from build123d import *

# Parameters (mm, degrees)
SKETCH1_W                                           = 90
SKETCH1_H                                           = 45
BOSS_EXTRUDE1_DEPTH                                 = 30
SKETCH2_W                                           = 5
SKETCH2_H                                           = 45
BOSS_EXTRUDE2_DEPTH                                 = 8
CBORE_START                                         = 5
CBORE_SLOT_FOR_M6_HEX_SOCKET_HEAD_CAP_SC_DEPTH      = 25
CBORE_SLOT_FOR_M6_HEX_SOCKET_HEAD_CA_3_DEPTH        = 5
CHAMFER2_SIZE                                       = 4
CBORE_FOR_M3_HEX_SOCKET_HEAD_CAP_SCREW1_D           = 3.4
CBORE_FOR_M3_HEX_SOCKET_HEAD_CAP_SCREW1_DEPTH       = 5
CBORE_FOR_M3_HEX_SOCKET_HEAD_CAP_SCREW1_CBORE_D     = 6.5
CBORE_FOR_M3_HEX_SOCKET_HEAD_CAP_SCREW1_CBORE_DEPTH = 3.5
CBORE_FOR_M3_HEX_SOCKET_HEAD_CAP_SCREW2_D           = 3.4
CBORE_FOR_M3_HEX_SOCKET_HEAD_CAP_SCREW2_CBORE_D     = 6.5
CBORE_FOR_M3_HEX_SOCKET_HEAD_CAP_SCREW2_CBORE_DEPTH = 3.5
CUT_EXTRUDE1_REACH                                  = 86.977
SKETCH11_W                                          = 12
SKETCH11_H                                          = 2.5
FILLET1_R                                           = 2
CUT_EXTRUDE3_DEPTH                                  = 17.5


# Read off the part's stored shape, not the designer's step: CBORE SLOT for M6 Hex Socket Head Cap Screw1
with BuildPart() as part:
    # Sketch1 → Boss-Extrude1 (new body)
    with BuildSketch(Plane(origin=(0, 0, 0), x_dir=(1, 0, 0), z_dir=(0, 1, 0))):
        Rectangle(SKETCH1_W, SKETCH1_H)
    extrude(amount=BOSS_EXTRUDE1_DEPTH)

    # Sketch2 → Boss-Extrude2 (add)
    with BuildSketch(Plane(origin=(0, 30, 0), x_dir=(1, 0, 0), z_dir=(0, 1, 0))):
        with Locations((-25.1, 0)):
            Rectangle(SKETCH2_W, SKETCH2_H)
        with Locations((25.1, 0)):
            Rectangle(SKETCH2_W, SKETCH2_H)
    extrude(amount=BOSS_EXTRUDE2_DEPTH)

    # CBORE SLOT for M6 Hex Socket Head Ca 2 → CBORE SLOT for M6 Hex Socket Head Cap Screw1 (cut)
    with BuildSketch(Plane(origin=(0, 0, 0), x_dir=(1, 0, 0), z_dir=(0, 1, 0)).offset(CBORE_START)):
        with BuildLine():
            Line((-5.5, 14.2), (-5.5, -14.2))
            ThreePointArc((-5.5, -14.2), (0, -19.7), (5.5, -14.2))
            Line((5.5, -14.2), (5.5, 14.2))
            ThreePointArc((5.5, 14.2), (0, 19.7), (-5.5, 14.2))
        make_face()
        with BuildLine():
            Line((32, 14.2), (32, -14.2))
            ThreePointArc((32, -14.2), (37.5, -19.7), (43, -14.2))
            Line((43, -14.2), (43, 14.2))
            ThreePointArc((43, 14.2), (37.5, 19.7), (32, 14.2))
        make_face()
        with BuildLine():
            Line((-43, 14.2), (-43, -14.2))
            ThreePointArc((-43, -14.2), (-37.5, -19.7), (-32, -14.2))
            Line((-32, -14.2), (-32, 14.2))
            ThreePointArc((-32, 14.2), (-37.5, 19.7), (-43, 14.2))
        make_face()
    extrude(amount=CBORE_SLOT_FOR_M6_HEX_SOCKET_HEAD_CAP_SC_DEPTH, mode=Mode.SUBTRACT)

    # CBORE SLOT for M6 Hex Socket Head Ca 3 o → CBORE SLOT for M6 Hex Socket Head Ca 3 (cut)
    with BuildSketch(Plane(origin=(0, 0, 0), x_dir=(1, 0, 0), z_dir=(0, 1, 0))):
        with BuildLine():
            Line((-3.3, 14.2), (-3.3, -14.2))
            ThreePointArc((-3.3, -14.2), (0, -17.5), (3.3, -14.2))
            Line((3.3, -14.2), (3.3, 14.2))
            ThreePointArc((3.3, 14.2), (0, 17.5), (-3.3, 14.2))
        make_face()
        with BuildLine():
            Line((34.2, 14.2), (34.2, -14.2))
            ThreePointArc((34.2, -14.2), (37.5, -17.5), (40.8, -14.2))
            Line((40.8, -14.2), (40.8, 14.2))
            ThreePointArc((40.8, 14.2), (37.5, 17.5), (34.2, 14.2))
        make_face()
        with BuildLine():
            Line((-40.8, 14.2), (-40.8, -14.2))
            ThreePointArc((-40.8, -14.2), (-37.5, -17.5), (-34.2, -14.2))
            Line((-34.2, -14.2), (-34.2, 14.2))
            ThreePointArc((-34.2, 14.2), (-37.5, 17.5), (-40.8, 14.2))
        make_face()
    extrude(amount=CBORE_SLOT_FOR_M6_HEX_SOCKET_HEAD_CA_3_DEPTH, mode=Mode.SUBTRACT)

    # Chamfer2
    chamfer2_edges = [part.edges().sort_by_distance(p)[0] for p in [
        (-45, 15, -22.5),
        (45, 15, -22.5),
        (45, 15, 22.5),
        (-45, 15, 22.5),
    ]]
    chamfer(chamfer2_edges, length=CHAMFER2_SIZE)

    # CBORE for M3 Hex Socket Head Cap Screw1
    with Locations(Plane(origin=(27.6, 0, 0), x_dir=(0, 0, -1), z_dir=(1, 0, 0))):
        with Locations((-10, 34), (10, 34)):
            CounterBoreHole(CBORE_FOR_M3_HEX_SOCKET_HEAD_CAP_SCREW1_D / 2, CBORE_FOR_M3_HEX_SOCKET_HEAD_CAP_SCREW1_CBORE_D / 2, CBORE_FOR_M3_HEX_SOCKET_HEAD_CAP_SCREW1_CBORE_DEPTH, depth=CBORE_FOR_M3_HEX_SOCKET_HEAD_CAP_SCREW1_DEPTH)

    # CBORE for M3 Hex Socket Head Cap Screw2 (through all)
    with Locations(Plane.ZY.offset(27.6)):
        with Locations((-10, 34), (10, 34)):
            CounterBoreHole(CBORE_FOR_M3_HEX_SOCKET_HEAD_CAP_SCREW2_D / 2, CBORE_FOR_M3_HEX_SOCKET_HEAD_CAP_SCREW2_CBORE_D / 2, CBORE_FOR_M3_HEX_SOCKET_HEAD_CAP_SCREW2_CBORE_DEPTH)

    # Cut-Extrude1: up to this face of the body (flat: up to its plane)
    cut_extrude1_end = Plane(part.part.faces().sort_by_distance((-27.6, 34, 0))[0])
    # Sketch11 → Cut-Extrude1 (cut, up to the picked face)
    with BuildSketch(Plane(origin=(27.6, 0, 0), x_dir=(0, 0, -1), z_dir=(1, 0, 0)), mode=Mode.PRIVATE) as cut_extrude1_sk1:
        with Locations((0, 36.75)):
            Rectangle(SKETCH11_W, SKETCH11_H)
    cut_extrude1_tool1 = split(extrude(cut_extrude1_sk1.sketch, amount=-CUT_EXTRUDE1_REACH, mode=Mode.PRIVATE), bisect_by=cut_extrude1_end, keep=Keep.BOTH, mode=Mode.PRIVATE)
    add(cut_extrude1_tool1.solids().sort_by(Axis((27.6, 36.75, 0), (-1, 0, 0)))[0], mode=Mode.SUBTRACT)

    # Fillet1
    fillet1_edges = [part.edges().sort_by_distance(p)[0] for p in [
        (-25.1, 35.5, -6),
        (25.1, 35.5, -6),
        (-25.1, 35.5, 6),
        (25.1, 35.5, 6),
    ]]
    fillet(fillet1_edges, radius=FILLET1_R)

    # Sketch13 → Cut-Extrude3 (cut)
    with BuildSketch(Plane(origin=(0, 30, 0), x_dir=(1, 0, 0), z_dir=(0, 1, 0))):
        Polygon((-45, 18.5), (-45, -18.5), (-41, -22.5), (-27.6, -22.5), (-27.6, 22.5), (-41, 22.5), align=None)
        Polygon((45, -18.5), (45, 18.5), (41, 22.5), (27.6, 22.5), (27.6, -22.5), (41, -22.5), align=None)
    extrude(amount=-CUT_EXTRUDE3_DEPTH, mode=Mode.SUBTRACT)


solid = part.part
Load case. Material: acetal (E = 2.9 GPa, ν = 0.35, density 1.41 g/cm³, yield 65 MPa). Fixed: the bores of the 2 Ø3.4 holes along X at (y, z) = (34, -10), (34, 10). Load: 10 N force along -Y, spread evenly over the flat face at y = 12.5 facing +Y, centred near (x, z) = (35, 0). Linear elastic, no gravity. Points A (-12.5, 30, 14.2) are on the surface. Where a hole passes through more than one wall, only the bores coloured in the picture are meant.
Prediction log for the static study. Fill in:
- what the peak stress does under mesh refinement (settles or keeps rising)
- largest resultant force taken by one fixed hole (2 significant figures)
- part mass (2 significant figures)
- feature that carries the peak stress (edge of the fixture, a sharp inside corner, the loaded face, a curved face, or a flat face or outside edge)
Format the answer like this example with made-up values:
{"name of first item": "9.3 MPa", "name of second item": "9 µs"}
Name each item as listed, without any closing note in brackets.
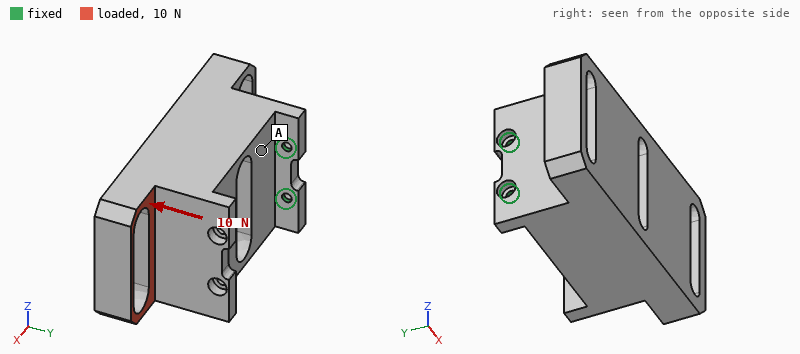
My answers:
{"what the peak stress does under mesh refinement": "keeps rising", "largest resultant force taken by one fixed hole": "5.0 N", "part mass": "110 g", "feature that carries the peak stress": "edge of the fixture"}
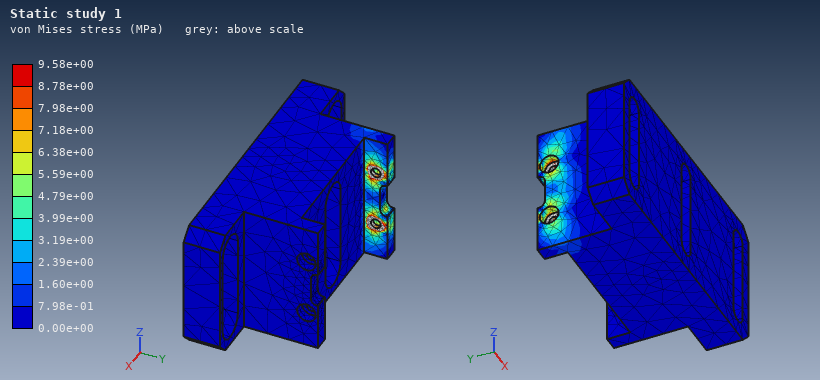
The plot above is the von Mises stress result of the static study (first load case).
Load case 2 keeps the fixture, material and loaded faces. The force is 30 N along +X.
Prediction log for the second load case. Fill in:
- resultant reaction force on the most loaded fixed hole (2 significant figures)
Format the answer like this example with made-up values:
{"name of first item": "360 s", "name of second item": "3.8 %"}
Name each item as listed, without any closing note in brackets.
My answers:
{"resultant reaction force on the most loaded fixed hole": "15 N"}
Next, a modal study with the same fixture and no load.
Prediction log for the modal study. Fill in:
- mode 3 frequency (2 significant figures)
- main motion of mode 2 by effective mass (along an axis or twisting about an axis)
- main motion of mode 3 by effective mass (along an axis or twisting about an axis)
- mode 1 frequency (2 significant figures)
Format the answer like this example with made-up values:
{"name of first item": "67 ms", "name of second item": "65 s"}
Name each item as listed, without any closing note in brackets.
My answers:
{"mode 3 frequency": "900 Hz", "main motion of mode 2 by effective mass": "along Z", "main motion of mode 3 by effective mass": "along Z", "mode 1 frequency": "77 Hz"}
